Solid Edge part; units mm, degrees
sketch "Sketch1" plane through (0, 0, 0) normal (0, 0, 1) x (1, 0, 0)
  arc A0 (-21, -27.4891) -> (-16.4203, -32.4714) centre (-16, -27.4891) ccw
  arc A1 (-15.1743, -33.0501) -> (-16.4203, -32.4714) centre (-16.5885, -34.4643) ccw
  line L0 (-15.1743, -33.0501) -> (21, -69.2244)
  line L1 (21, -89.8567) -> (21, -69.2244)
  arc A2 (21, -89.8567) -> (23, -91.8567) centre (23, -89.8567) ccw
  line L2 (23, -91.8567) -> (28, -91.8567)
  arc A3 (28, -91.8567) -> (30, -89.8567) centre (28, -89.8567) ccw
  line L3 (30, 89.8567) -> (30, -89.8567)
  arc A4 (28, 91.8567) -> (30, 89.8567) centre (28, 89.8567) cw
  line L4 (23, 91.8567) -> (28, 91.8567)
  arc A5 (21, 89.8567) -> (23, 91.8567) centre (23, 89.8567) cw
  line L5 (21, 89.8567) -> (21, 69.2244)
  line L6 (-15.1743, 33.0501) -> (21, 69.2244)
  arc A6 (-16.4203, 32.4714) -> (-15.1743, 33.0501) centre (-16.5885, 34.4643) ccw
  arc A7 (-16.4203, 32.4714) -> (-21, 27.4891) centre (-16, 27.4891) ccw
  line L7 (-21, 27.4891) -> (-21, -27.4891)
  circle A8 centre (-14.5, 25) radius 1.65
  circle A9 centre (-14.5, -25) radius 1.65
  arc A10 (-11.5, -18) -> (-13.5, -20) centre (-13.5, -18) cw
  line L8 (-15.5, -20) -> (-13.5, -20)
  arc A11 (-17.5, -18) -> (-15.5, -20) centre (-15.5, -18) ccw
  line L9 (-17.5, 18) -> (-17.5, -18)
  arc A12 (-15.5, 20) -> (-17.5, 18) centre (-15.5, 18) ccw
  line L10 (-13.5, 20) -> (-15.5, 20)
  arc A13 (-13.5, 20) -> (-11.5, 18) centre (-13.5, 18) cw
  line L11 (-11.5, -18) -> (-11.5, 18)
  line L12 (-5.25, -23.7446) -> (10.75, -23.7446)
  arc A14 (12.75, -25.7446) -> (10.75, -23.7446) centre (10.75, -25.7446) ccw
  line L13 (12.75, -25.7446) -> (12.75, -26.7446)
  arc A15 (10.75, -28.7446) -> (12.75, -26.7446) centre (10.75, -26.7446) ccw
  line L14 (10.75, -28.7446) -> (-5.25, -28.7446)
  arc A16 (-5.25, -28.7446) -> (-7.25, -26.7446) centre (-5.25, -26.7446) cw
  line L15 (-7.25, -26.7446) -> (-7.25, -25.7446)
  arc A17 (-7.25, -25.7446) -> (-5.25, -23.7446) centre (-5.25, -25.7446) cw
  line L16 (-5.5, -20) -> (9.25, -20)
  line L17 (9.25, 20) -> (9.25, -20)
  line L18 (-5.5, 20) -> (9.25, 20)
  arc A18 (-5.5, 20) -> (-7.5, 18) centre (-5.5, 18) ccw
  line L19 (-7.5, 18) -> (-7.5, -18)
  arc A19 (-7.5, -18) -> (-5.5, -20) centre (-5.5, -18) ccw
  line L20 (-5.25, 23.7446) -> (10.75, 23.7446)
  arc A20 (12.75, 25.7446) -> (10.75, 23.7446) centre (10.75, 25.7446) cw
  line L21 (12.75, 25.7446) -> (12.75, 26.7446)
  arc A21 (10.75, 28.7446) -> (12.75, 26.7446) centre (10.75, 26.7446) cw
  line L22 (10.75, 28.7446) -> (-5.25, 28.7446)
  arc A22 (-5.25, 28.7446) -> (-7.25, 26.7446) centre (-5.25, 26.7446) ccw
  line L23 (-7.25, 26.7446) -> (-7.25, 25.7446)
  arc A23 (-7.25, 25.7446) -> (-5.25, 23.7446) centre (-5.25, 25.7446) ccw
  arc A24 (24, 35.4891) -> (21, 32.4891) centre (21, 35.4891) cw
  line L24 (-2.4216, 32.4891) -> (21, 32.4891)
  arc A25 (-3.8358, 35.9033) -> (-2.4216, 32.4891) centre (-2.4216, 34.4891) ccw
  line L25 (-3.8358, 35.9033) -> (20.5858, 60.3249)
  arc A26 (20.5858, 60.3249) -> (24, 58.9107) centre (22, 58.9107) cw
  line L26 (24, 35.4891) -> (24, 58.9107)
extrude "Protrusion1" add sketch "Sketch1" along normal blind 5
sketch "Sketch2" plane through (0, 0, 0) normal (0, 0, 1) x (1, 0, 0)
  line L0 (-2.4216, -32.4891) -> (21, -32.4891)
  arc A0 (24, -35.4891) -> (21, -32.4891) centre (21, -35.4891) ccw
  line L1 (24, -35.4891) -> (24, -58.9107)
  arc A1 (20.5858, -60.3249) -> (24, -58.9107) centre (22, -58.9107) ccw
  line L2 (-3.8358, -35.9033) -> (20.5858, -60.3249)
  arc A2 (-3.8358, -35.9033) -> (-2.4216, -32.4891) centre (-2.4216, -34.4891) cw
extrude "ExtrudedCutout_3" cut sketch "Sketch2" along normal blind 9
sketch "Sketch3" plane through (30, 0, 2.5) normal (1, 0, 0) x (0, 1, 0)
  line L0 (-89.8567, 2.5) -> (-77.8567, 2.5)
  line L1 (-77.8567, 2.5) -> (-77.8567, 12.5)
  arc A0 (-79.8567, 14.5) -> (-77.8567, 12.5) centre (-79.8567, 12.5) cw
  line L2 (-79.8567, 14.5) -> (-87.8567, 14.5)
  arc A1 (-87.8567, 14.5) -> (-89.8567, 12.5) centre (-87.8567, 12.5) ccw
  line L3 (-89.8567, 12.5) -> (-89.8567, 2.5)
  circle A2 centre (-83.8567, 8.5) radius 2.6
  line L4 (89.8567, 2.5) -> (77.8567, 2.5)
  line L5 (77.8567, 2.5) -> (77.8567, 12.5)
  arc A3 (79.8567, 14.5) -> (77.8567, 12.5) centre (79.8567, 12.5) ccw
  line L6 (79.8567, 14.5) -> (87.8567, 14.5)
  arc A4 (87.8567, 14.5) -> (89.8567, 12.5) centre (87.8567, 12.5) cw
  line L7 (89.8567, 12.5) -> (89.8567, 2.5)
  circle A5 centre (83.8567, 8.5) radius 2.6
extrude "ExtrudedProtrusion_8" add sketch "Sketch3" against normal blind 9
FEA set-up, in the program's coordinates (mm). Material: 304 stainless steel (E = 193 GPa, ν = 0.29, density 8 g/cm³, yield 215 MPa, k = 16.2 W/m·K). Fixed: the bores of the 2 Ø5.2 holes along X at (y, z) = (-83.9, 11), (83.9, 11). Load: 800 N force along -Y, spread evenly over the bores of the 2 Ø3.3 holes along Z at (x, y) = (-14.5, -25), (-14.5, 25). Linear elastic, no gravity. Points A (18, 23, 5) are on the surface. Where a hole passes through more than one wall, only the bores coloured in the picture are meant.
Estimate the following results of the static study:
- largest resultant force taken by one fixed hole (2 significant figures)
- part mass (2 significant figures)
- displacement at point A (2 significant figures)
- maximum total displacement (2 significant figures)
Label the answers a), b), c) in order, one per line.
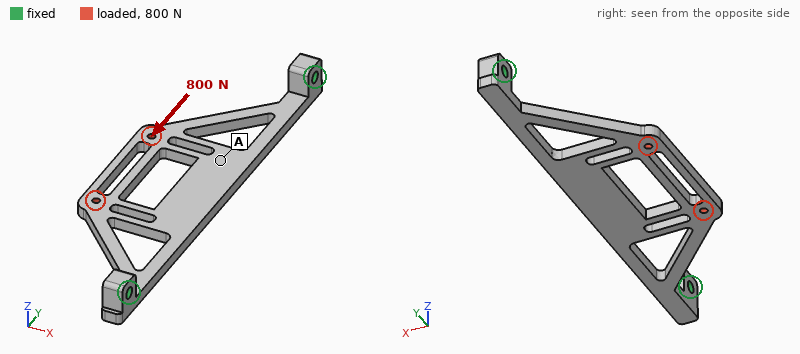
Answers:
a) 450 N
b) 160 g
c) 4.0 µm
d) 14 µm
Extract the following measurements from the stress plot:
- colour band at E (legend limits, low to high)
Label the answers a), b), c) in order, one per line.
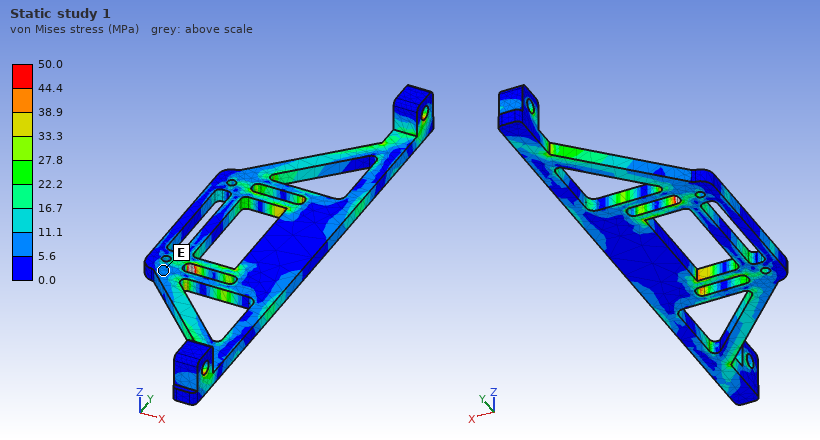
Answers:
a) 5.6 to 11.1 MPa
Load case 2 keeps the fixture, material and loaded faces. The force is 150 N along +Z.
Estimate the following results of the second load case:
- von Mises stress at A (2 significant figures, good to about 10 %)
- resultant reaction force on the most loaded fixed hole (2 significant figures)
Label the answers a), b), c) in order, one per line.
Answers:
a) 18 MPa
b) 99 N
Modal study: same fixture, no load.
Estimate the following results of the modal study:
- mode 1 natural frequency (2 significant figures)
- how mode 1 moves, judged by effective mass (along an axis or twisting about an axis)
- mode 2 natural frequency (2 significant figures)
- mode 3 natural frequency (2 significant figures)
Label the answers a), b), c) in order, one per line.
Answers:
a) 530 Hz
b) along Z
c) 1100 Hz
d) 1700 Hz
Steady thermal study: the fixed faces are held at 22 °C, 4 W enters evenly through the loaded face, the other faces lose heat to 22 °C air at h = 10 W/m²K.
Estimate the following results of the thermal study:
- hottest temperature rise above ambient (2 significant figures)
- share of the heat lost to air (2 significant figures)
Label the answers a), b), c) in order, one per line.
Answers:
a) 61 K
b) 80 %
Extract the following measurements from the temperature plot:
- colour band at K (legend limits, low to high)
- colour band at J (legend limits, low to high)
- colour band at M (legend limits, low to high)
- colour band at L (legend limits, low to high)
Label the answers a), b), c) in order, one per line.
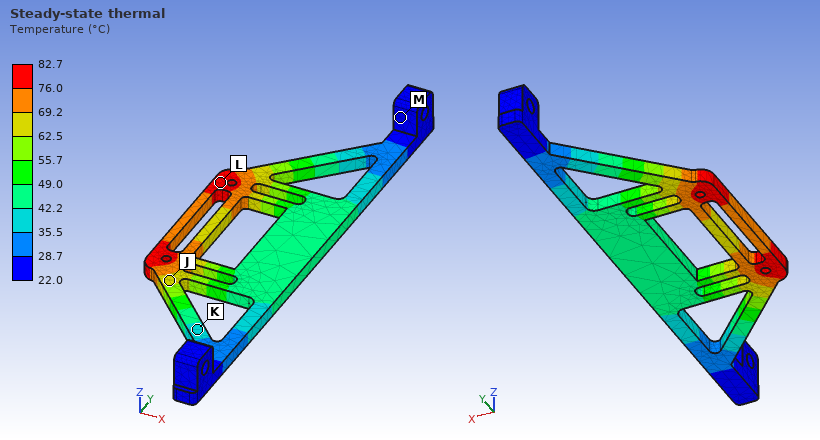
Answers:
a) 35.5 to 42.2 °C
b) 62.5 to 69.2 °C
c) 22.0 to 28.7 °C
d) 76.0 to 82.7 °C
